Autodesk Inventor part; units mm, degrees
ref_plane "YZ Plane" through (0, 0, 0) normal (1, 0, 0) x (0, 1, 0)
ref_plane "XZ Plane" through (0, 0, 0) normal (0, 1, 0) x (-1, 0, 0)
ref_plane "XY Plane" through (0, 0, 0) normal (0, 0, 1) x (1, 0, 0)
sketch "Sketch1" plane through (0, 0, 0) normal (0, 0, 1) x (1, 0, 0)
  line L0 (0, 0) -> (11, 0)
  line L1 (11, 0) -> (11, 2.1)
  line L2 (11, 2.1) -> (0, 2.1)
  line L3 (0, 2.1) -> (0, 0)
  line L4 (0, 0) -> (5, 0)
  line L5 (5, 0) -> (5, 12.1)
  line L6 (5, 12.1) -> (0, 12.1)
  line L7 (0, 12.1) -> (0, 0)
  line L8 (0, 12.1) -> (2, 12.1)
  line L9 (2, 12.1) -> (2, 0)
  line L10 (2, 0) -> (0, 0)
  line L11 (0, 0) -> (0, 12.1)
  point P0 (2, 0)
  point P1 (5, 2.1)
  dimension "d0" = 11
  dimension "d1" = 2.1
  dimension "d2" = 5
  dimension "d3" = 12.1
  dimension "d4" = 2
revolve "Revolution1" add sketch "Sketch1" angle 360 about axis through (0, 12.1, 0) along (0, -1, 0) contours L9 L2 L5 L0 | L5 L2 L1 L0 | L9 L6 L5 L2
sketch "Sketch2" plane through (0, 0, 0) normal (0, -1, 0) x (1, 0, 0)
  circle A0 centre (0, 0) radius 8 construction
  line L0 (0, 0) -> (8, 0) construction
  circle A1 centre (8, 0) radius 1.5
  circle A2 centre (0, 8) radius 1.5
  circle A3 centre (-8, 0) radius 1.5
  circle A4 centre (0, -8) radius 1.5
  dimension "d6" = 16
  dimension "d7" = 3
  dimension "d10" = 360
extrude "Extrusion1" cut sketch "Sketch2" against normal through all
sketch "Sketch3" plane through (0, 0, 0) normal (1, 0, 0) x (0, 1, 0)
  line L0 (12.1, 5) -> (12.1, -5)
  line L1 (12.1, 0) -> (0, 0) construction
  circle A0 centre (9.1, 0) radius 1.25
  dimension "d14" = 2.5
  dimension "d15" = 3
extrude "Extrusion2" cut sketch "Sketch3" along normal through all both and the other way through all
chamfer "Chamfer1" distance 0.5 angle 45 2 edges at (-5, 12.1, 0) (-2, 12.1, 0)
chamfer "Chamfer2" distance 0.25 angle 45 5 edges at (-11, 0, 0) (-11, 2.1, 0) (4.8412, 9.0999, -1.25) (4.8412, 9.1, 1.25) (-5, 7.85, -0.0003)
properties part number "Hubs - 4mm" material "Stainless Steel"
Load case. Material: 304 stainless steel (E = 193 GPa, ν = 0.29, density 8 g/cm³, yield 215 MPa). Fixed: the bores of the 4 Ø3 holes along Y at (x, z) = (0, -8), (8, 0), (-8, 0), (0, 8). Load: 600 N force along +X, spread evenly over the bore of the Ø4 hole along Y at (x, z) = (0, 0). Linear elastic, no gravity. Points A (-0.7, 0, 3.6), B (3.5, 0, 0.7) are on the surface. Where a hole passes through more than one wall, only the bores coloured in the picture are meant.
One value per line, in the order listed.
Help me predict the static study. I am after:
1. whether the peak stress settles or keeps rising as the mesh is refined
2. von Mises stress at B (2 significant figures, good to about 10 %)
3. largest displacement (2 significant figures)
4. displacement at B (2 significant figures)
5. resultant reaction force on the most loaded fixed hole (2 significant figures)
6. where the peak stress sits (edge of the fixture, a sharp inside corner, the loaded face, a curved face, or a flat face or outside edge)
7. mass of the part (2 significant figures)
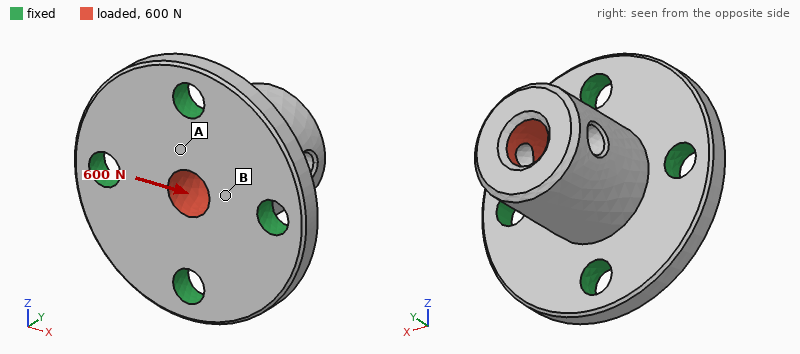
keeps rising
11 MPa
3.6 µm
0.67 µm
290 N
edge of the fixture
11 g
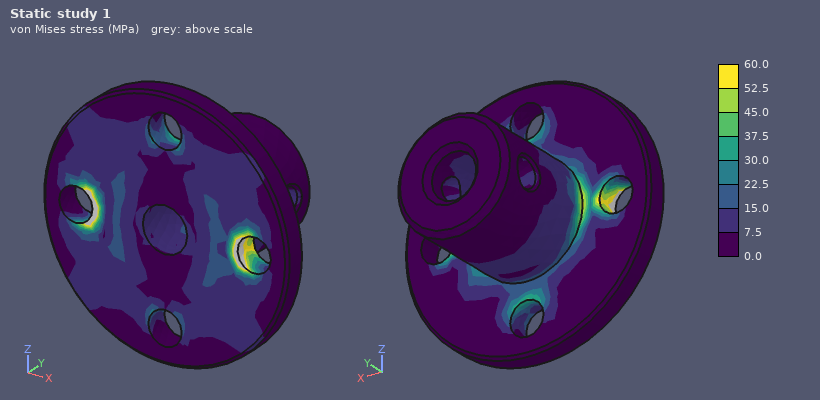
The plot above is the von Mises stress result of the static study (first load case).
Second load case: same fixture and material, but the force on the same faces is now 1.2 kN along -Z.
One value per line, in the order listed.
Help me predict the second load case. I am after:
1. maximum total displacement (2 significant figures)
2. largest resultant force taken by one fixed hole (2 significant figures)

7.4 µm
580 N
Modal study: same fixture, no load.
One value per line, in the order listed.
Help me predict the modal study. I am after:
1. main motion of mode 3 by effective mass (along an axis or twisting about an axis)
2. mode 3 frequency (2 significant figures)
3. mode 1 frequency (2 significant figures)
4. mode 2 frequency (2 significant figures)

along Y
49 kHz
29 kHz
30 kHz
